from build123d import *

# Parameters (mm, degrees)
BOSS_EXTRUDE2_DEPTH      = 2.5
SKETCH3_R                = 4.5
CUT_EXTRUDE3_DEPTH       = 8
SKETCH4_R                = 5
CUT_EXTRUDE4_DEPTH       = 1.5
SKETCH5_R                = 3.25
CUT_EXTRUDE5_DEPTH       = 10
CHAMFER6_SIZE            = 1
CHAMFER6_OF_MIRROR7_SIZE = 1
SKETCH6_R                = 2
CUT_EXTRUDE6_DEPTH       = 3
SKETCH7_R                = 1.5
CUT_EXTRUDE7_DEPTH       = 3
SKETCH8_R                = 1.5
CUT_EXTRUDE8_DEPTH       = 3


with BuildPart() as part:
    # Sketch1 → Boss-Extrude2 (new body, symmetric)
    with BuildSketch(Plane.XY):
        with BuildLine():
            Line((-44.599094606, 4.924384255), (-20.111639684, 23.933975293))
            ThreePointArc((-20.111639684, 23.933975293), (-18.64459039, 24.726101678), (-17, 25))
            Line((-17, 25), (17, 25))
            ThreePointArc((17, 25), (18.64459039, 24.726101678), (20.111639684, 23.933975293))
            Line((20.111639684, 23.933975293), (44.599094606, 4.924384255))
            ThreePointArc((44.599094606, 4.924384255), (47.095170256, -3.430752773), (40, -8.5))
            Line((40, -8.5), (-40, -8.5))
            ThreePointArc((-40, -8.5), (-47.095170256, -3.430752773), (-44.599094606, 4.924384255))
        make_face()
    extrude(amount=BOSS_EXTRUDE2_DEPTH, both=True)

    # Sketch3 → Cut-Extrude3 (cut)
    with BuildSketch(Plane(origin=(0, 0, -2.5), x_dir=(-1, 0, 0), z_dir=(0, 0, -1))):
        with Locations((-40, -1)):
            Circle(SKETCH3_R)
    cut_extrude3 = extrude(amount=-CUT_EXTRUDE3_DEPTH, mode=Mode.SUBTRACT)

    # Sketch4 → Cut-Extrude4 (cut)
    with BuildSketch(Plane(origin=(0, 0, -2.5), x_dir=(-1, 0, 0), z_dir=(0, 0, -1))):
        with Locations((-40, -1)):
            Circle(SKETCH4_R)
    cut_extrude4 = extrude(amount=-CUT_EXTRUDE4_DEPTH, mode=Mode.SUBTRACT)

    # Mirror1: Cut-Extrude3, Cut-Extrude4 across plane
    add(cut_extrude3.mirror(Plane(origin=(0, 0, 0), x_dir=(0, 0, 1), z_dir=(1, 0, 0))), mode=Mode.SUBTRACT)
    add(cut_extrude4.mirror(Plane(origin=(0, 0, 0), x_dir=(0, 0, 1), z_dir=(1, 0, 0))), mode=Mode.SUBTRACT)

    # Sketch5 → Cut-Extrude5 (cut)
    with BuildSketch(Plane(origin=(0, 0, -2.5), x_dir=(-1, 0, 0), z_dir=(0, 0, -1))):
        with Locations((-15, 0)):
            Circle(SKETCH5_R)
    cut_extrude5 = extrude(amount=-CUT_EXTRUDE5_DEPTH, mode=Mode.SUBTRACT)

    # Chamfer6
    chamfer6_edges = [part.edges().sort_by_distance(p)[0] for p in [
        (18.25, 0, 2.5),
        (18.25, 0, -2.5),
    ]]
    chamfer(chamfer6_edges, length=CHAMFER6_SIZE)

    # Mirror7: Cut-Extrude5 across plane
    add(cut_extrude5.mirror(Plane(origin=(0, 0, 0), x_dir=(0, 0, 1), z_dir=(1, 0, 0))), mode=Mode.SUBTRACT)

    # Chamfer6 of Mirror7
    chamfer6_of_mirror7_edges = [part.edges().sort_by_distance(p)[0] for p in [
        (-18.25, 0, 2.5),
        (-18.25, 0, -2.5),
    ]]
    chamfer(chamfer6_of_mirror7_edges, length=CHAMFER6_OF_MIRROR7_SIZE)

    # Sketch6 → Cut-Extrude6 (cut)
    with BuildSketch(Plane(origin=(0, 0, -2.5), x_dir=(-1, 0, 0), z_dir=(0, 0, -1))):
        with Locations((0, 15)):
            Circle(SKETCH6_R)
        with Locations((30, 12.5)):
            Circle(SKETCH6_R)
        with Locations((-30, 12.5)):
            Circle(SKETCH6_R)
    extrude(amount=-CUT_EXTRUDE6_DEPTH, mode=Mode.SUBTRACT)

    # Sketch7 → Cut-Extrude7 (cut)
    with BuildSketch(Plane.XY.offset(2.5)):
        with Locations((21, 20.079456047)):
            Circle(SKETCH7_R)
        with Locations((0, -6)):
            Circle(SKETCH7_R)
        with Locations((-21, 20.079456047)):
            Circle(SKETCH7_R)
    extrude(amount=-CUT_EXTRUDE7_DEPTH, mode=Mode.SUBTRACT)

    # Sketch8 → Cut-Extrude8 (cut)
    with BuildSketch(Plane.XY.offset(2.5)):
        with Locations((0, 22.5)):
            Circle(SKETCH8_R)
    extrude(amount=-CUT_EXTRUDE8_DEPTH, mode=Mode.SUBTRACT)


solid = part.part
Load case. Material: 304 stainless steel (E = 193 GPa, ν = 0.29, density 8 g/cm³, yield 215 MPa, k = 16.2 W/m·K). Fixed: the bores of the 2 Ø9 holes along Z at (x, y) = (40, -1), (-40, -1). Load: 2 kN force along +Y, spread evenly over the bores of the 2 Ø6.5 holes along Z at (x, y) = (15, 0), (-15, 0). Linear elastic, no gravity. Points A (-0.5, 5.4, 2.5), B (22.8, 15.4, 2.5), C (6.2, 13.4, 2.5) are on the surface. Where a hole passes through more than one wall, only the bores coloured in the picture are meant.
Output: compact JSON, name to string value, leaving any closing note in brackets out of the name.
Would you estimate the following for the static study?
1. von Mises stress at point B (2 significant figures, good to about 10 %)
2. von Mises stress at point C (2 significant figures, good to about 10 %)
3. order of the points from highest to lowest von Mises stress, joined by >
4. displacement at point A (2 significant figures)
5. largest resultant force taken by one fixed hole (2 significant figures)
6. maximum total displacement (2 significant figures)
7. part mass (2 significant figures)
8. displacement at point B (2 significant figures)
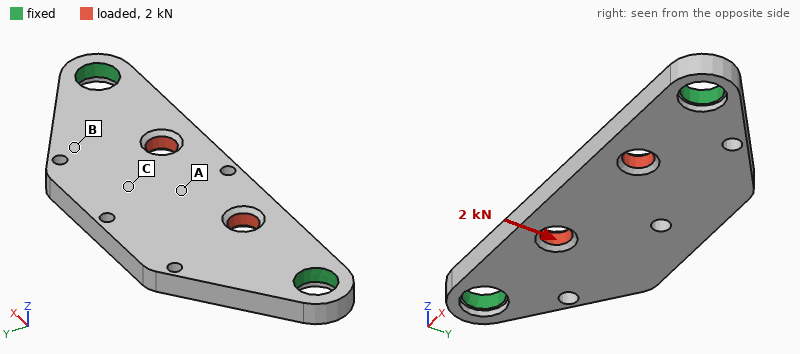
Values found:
{"von Mises stress at point B": "15 MPa", "von Mises stress at point C": "10 MPa", "order of the points from highest to lowest von Mises stress, joined by >": "B > C > A", "displacement at point A": "5.6 µm", "largest resultant force taken by one fixed hole": "1.1 kN", "maximum total displacement": "6.0 µm", "part mass": "90 g", "displacement at point B": "3.8 µm"}
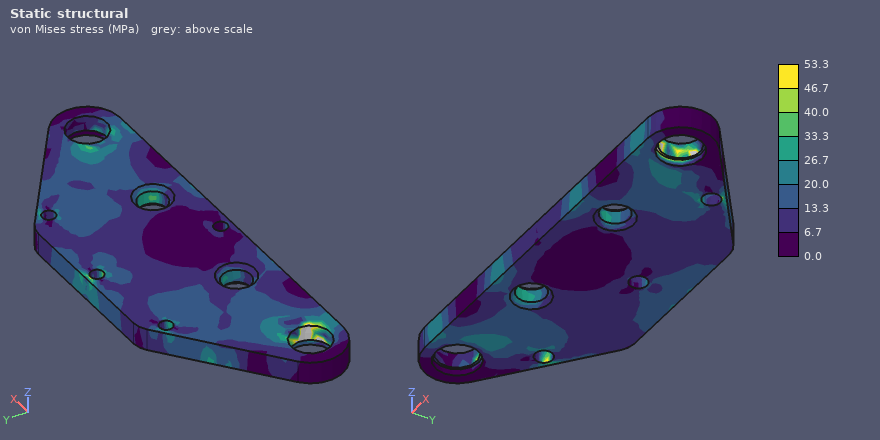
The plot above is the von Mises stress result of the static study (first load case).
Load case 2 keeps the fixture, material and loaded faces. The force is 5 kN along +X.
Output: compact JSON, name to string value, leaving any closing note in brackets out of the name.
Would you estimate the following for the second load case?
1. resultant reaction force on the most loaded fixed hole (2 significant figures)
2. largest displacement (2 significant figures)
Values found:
{"resultant reaction force on the most loaded fixed hole": "2.5 kN", "largest displacement": "4.9 µm"}
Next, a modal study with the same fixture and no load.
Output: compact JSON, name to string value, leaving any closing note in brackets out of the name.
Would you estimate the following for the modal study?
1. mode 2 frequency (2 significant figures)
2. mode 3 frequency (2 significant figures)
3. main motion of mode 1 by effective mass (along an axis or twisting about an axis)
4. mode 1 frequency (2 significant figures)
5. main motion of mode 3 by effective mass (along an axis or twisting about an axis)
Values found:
{"mode 2 frequency": "5600 Hz", "mode 3 frequency": "8100 Hz", "main motion of mode 1 by effective mass": "along Z", "mode 1 frequency": "2900 Hz", "main motion of mode 3 by effective mass": "twisting about Y"}
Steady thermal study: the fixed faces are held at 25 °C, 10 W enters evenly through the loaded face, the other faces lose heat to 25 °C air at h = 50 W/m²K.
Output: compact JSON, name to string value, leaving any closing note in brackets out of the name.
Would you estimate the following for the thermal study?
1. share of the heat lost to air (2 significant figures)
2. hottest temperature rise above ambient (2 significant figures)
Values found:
{"share of the heat lost to air": "57 %", "hottest temperature rise above ambient": "43 K"}
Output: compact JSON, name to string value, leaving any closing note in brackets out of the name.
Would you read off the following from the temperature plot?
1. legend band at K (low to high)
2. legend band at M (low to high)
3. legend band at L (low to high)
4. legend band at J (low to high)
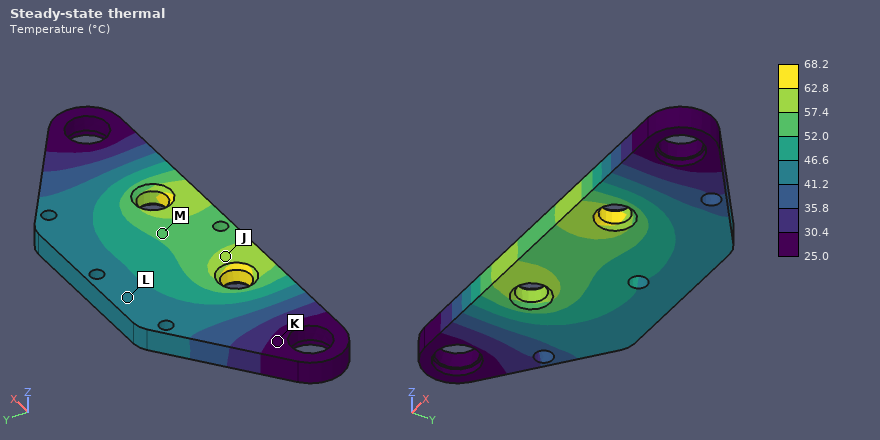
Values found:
{"legend band at K": "25.0 to 30.4 °C", "legend band at M": "52.0 to 57.4 °C", "legend band at L": "41.2 to 46.6 °C", "legend band at J": "57.4 to 62.8 °C"}
